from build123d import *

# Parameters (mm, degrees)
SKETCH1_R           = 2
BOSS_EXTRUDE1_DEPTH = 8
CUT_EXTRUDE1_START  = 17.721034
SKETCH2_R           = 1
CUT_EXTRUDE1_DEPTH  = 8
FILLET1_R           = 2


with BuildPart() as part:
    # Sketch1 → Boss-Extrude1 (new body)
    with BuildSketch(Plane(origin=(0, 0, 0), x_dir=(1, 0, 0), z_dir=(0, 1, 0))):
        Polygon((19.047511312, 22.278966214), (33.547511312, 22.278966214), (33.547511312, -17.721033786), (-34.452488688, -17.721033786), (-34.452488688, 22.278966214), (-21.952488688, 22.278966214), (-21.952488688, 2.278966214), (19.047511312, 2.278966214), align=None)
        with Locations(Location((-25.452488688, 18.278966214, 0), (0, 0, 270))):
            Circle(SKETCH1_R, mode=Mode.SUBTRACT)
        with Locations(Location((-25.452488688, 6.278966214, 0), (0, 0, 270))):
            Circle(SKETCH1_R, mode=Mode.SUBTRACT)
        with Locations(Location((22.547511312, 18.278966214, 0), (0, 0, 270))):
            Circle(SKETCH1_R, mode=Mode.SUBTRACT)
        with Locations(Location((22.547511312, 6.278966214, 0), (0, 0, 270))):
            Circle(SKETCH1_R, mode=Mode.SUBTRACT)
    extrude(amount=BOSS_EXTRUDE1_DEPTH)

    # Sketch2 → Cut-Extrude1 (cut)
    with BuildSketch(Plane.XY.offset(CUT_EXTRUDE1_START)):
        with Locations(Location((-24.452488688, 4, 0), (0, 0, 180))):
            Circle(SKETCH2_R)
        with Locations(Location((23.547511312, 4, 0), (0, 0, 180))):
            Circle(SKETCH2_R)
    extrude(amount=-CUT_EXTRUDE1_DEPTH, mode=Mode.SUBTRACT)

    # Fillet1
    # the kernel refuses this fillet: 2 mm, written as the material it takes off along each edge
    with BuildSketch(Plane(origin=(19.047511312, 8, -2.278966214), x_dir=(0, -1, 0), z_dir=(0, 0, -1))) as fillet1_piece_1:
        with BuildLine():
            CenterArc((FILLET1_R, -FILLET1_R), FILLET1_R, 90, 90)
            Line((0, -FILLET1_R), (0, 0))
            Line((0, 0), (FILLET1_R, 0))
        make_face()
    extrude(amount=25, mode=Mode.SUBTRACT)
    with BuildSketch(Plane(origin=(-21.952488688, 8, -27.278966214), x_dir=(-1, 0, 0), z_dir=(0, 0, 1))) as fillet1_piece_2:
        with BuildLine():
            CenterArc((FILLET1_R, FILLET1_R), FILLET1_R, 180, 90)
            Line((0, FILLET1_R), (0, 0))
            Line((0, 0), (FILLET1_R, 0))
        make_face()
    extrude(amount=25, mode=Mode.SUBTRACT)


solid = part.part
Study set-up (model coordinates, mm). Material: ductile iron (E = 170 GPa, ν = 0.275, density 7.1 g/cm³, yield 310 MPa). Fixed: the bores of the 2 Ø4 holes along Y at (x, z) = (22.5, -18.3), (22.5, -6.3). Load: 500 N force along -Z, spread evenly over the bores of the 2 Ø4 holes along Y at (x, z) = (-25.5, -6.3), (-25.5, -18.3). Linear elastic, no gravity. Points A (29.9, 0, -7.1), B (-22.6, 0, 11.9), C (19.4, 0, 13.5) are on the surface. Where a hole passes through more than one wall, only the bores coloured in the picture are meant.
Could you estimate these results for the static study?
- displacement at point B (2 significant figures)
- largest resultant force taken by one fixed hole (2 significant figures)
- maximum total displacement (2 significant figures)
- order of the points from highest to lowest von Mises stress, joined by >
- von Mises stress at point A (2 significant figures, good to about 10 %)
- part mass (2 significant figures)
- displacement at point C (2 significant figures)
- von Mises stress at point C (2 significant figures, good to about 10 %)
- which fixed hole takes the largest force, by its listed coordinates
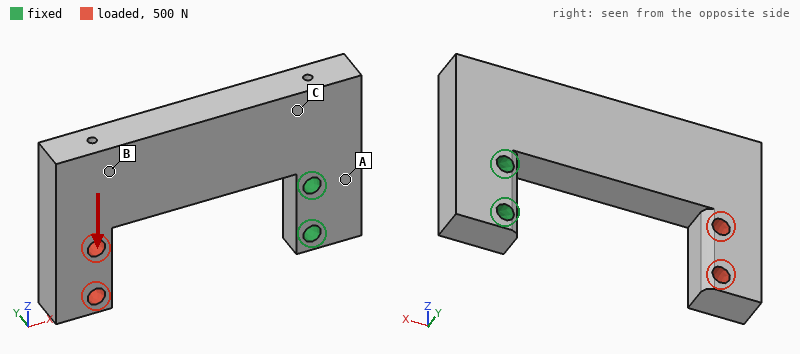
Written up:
0.075 mm
2.0 kN
0.10 mm
A > C > B
41 MPa
100 g
0.020 mm
24 MPa
(22.5, -6.3)
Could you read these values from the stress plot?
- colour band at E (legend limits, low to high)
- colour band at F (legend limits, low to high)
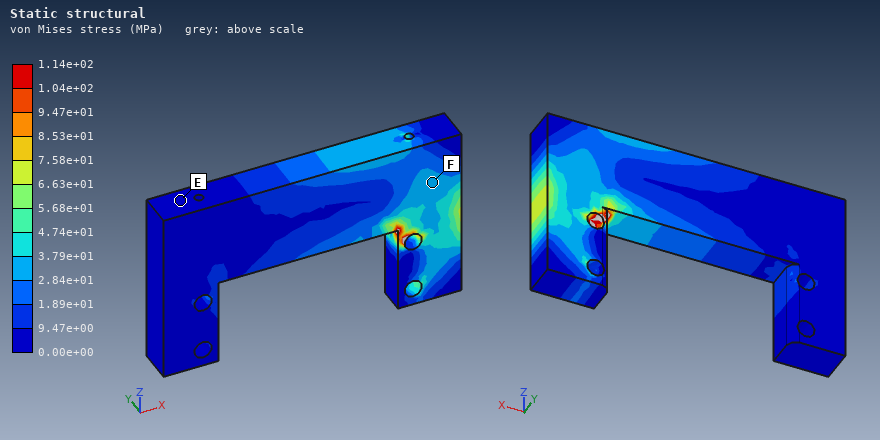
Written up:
0.00e+00 to 9.47e+00 MPa
2.84e+01 to 3.79e+01 MPa
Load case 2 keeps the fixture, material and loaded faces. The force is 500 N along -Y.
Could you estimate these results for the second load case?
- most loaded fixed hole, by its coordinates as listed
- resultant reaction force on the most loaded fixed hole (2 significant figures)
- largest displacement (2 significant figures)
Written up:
(22.5, -6.3)
380 N
0.39 mm
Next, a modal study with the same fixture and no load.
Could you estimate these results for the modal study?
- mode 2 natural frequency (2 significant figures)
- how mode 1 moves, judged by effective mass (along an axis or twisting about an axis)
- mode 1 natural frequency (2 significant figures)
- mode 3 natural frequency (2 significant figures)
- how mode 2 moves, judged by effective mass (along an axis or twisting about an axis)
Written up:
1800 Hz
along Y
1100 Hz
3200 Hz
along Z
